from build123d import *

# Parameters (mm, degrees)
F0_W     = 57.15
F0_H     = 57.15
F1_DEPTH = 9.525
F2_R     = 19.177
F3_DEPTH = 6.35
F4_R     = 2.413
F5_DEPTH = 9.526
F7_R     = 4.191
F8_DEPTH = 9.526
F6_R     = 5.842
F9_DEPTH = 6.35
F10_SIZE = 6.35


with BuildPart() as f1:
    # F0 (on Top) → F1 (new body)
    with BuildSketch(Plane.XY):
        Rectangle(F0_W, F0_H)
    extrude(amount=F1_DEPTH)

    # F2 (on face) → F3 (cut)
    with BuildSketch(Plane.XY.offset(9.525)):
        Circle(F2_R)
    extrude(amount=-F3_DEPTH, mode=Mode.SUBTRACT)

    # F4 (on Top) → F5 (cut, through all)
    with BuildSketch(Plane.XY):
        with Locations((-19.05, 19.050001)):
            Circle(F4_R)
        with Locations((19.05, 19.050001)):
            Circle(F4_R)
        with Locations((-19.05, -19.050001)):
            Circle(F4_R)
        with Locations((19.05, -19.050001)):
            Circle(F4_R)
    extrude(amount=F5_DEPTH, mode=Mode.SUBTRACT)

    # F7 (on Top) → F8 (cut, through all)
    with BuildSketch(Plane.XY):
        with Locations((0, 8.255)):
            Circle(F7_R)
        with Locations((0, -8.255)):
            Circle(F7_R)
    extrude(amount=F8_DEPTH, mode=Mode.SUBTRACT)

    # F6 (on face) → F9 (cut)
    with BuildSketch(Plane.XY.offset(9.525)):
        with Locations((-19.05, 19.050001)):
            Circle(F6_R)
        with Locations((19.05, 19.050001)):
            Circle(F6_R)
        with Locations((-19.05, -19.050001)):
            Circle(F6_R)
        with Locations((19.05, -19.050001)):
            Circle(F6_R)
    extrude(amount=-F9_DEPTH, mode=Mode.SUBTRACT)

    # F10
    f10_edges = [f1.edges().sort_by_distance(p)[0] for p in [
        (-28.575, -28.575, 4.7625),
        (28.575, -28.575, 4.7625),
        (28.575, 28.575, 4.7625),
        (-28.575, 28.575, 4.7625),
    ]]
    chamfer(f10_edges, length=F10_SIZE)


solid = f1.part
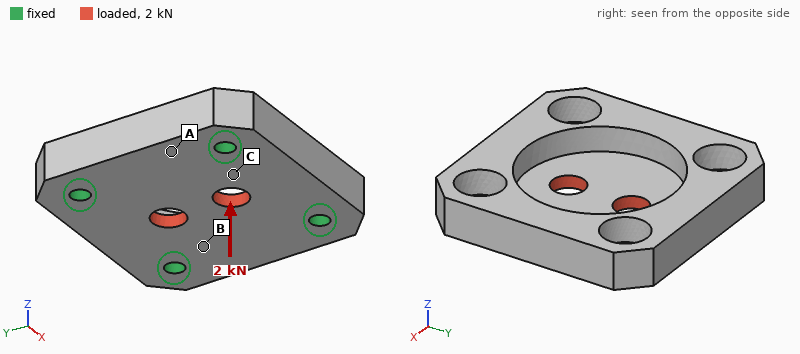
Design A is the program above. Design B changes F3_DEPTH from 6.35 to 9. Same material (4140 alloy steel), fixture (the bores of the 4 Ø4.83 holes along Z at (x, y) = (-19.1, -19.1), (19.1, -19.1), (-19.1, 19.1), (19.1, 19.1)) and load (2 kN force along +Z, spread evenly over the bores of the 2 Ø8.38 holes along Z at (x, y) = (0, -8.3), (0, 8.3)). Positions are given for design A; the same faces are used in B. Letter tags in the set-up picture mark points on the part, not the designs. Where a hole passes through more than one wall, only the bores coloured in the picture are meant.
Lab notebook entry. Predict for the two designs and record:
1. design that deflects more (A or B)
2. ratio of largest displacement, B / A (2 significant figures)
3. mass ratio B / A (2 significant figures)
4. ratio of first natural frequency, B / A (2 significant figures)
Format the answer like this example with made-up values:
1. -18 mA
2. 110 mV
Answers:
1. B
2. 110
3. 0.86
4. 0.29
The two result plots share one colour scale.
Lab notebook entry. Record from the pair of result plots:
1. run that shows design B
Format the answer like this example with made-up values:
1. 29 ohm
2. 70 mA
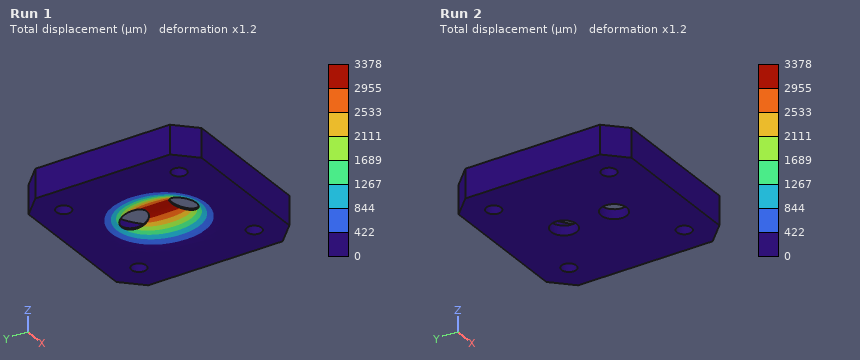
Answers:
1. Run 1
